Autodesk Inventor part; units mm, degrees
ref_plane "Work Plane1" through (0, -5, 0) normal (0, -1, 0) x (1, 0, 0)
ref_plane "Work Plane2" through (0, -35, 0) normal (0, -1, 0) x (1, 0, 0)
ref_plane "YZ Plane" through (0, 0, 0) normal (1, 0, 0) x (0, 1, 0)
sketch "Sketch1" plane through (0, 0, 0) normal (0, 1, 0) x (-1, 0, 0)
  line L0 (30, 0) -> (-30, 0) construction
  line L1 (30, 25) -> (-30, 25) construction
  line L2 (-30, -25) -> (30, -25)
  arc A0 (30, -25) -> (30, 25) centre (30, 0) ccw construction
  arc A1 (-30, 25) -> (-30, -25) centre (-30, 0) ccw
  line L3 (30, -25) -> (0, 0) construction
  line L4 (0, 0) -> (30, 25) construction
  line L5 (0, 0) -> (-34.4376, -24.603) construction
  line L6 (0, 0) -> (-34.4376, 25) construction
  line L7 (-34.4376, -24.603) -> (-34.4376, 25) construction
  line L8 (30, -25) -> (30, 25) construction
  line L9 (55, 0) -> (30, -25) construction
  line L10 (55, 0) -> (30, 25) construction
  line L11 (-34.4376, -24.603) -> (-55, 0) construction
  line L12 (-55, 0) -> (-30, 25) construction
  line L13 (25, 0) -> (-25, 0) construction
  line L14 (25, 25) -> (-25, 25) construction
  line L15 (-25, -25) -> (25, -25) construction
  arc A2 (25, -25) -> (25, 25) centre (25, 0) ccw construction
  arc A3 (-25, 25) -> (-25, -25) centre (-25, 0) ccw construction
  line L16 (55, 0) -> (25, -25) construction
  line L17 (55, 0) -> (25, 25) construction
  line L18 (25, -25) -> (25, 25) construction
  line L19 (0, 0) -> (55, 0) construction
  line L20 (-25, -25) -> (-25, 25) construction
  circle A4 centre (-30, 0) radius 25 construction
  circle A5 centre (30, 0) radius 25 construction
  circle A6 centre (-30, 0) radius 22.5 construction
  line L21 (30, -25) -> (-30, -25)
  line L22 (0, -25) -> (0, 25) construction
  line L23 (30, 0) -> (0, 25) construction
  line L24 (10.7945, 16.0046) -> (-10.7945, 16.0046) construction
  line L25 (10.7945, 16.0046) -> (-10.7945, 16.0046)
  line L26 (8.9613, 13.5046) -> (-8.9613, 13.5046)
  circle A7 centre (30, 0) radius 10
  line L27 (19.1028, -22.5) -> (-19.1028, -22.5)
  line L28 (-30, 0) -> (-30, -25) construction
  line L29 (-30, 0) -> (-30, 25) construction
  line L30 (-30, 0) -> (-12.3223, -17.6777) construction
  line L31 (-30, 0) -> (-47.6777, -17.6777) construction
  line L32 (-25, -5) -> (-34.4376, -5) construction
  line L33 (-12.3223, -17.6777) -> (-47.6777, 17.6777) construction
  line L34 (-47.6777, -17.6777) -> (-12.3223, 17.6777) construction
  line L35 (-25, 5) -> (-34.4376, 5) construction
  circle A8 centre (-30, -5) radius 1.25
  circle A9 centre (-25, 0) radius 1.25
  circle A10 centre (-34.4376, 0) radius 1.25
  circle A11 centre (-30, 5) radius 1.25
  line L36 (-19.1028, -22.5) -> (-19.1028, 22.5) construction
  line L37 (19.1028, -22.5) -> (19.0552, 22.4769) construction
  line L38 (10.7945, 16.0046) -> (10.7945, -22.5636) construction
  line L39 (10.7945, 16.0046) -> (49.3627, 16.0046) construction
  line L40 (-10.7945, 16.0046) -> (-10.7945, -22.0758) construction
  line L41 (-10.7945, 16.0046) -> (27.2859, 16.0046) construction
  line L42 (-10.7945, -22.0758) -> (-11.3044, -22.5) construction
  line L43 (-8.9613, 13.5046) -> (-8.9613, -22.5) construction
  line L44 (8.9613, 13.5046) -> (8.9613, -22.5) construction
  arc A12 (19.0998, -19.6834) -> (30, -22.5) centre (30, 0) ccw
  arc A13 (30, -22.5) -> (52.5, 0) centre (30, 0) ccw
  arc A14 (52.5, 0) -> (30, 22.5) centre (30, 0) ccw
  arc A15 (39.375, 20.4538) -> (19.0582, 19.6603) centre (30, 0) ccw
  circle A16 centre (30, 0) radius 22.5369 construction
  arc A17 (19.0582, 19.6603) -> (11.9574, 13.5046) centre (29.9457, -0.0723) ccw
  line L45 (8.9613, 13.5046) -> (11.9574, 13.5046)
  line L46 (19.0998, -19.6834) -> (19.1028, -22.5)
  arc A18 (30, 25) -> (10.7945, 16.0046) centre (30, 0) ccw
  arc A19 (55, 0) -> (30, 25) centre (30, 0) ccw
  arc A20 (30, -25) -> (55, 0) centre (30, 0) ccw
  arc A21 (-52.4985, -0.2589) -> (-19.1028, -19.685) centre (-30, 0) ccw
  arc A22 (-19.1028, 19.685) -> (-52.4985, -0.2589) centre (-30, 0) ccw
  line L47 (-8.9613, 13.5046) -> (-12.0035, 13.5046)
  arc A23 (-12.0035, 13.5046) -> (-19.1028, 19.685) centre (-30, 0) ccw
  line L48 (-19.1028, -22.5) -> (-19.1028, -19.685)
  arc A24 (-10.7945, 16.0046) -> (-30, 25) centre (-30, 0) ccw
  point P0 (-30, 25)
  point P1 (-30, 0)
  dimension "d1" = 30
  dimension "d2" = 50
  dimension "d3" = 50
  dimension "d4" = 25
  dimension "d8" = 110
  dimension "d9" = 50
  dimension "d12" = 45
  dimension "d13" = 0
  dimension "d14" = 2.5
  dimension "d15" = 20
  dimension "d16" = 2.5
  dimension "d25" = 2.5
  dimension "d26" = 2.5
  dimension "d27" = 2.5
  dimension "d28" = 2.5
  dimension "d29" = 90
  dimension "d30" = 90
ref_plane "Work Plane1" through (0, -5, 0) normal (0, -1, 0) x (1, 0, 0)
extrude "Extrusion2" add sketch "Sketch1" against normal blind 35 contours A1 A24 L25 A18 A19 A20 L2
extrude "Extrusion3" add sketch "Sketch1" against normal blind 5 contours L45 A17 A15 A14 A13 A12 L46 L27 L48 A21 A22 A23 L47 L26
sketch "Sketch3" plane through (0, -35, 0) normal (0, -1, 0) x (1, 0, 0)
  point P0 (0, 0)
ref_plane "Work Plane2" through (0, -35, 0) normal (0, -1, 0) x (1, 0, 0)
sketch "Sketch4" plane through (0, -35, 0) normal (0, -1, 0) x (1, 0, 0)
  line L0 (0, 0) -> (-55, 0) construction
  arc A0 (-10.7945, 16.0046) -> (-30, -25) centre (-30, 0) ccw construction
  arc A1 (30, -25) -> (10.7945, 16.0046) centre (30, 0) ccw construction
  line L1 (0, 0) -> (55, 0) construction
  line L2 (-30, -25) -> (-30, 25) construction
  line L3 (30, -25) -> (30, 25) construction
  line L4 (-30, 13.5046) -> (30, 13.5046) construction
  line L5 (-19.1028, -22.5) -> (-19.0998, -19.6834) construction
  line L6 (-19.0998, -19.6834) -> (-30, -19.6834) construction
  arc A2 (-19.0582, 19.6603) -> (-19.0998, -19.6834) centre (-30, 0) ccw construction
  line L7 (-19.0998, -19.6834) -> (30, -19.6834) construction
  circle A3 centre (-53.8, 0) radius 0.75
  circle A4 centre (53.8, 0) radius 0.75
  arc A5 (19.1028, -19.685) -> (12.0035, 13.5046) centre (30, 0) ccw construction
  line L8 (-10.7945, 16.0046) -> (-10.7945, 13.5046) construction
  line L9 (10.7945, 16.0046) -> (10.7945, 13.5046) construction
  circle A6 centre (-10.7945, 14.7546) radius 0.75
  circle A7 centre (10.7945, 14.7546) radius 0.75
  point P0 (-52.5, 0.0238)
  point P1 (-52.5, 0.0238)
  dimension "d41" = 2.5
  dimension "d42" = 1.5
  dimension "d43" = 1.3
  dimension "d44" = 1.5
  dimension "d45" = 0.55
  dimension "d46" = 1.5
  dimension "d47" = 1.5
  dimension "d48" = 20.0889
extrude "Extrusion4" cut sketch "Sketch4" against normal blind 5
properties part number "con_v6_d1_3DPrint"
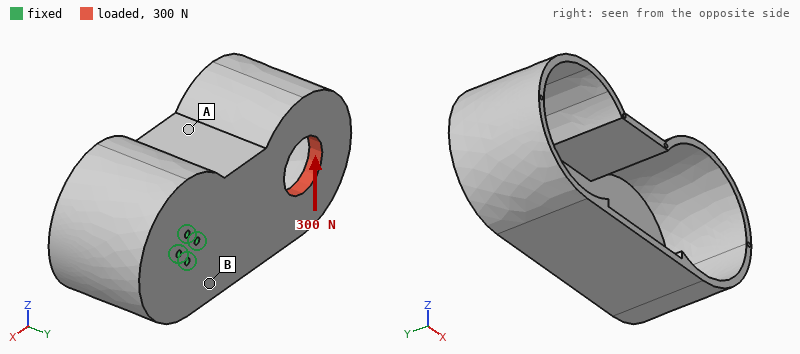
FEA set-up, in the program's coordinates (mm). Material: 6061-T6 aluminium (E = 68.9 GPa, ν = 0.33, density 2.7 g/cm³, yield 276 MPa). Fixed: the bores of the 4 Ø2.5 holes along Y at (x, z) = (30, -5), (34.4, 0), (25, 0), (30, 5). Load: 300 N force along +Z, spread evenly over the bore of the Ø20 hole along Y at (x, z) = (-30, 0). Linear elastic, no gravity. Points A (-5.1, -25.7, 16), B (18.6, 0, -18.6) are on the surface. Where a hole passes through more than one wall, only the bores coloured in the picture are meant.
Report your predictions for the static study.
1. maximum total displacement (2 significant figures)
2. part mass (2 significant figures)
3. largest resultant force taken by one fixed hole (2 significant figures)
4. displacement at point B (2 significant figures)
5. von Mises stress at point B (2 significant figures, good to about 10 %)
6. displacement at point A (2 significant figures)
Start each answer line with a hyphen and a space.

- 49 µm
- 120 g
- 870 N
- 8.6 µm
- 4.9 MPa
- 18 µm
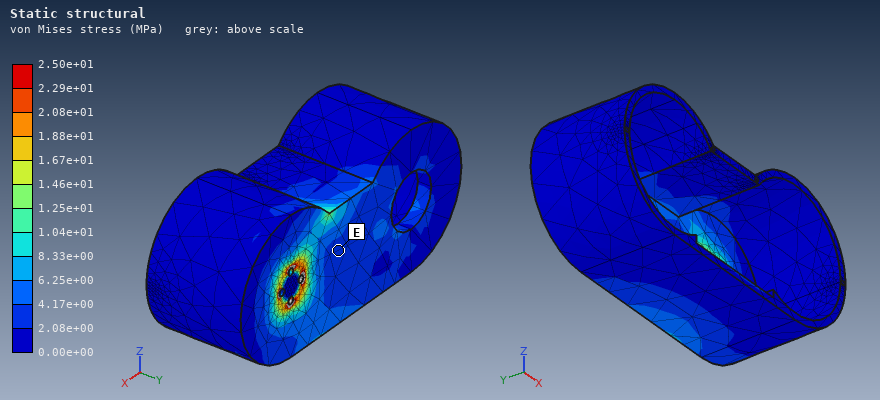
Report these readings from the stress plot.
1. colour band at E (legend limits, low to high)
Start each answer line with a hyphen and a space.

- 2.08e+00 to 4.17e+00 MPa
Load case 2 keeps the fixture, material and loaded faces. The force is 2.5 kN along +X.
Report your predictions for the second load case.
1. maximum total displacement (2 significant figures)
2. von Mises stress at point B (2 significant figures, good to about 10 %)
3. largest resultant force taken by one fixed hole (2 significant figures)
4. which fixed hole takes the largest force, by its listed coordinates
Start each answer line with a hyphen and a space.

- 27 µm
- 5.6 MPa
- 830 N
- (25, 0)
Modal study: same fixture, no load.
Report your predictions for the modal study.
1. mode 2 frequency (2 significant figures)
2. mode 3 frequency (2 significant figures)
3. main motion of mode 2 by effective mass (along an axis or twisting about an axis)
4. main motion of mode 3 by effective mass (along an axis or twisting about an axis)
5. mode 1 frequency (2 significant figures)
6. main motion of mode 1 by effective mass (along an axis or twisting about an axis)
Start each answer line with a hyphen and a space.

- 1100 Hz
- 2100 Hz
- along Z
- along Z
- 800 Hz
- along Y
